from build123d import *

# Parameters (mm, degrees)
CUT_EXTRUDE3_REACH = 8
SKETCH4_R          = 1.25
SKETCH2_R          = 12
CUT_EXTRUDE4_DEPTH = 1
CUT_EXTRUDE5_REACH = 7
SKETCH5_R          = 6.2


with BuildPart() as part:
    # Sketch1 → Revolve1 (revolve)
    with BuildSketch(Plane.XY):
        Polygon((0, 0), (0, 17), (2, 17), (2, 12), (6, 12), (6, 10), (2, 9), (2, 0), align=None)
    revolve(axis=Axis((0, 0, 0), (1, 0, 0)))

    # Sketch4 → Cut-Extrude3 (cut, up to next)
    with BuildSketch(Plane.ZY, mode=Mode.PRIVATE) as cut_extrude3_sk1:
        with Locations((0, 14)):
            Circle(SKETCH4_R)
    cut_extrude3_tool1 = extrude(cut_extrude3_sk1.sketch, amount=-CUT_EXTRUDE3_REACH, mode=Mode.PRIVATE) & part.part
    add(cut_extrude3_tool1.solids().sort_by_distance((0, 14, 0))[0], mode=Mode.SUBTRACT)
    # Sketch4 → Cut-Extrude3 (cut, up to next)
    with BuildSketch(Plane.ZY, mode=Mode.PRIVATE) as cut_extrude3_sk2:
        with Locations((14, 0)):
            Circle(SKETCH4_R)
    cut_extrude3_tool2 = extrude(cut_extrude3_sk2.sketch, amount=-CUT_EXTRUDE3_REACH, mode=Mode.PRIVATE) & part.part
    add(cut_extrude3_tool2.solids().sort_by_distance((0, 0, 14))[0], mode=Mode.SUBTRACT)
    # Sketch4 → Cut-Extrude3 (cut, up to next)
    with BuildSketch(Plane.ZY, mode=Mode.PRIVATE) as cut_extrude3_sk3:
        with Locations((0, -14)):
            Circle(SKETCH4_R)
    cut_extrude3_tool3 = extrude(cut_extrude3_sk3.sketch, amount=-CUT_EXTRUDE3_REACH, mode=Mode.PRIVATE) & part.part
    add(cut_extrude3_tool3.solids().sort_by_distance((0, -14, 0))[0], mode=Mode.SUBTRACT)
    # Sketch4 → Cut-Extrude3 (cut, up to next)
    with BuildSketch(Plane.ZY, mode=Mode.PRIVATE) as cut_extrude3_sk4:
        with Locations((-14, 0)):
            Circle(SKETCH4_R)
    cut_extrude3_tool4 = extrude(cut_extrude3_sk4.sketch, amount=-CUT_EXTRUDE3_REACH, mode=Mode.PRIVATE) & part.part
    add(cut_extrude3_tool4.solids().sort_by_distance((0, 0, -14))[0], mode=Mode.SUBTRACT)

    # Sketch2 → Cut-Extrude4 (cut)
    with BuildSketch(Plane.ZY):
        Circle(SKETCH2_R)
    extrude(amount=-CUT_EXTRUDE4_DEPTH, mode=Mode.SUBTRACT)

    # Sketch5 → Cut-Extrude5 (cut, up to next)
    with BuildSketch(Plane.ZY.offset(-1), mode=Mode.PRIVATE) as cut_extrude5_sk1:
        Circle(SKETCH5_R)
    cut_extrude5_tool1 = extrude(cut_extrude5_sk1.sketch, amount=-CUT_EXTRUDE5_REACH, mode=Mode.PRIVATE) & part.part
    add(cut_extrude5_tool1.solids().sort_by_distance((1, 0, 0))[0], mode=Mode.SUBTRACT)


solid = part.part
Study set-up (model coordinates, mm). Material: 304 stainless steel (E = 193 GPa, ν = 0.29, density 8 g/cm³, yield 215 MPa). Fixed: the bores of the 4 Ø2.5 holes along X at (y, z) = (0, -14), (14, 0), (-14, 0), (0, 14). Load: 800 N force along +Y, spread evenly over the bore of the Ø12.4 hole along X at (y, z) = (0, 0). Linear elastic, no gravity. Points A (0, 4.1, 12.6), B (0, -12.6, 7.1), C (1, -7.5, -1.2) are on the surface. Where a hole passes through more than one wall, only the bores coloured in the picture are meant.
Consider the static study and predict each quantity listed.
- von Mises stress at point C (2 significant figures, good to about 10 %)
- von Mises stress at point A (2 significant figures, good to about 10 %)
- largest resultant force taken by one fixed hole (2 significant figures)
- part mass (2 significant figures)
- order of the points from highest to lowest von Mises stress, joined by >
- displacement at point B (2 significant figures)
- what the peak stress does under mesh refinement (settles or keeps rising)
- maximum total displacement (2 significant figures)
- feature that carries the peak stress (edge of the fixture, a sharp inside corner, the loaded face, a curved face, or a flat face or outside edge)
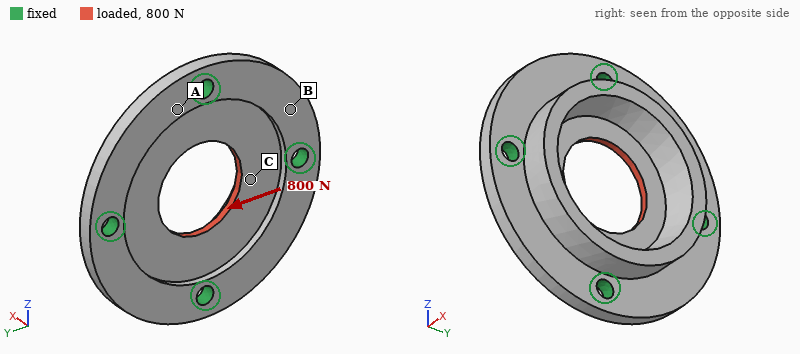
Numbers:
25 MPa
9.1 MPa
210 N
15 g
C > A > B
0.46 µm
keeps rising
1.3 µm
edge of the fixture
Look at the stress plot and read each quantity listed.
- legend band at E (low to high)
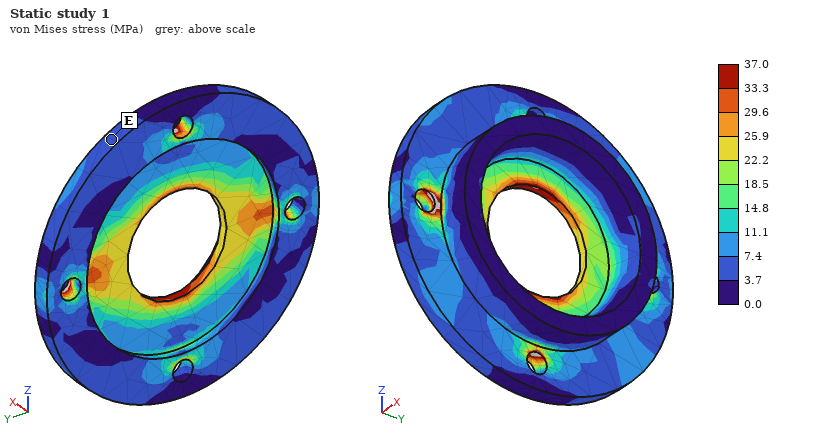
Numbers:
3.7 to 7.4 MPa
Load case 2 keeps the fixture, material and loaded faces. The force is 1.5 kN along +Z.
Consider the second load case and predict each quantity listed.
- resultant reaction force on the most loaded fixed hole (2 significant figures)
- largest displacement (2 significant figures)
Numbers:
400 N
2.4 µm
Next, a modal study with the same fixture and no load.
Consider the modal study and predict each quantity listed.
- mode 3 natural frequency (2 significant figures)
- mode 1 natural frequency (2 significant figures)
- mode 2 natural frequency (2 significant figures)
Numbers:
25 kHz
22 kHz
25 kHz
